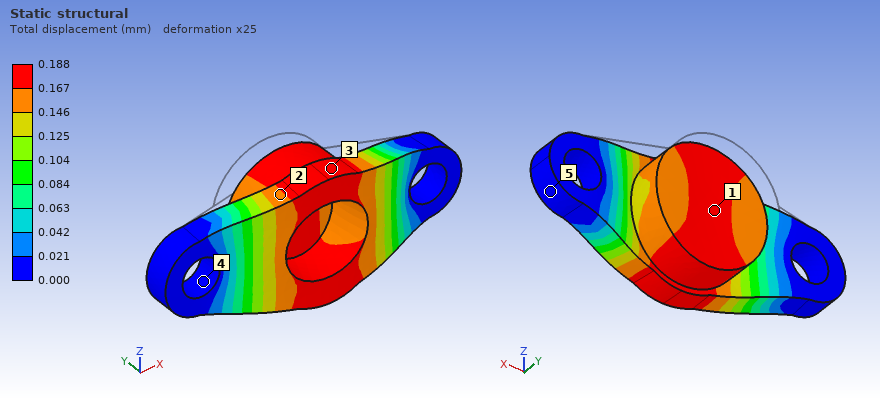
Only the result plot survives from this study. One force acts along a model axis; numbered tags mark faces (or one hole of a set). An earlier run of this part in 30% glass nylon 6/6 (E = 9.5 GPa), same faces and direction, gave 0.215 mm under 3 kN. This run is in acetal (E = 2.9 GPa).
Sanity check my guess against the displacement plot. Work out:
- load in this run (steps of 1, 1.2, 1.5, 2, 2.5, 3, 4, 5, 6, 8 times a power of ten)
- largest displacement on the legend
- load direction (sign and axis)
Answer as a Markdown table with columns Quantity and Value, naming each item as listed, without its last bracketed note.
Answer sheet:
| Quantity | Value |
|---|---|
| load in this run | 800 N |
| largest displacement on the legend | 0.188 mm |
| load direction | -Y |
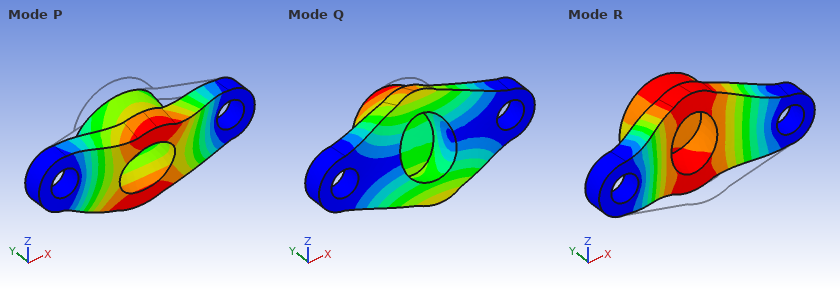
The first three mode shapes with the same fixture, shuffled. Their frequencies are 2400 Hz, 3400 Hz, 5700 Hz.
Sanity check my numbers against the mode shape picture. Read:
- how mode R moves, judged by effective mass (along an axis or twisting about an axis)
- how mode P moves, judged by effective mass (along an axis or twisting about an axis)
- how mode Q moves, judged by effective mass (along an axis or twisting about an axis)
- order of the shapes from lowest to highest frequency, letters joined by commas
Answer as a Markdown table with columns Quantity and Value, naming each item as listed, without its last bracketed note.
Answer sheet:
| Quantity | Value |
|---|---|
| how mode R moves, judged by effective mass | along Y |
| how mode P moves, judged by effective mass | along Z |
| how mode Q moves, judged by effective mass | along Z |
| order of the shapes from lowest to highest frequency, letters joined by commas | Q, R, P |
